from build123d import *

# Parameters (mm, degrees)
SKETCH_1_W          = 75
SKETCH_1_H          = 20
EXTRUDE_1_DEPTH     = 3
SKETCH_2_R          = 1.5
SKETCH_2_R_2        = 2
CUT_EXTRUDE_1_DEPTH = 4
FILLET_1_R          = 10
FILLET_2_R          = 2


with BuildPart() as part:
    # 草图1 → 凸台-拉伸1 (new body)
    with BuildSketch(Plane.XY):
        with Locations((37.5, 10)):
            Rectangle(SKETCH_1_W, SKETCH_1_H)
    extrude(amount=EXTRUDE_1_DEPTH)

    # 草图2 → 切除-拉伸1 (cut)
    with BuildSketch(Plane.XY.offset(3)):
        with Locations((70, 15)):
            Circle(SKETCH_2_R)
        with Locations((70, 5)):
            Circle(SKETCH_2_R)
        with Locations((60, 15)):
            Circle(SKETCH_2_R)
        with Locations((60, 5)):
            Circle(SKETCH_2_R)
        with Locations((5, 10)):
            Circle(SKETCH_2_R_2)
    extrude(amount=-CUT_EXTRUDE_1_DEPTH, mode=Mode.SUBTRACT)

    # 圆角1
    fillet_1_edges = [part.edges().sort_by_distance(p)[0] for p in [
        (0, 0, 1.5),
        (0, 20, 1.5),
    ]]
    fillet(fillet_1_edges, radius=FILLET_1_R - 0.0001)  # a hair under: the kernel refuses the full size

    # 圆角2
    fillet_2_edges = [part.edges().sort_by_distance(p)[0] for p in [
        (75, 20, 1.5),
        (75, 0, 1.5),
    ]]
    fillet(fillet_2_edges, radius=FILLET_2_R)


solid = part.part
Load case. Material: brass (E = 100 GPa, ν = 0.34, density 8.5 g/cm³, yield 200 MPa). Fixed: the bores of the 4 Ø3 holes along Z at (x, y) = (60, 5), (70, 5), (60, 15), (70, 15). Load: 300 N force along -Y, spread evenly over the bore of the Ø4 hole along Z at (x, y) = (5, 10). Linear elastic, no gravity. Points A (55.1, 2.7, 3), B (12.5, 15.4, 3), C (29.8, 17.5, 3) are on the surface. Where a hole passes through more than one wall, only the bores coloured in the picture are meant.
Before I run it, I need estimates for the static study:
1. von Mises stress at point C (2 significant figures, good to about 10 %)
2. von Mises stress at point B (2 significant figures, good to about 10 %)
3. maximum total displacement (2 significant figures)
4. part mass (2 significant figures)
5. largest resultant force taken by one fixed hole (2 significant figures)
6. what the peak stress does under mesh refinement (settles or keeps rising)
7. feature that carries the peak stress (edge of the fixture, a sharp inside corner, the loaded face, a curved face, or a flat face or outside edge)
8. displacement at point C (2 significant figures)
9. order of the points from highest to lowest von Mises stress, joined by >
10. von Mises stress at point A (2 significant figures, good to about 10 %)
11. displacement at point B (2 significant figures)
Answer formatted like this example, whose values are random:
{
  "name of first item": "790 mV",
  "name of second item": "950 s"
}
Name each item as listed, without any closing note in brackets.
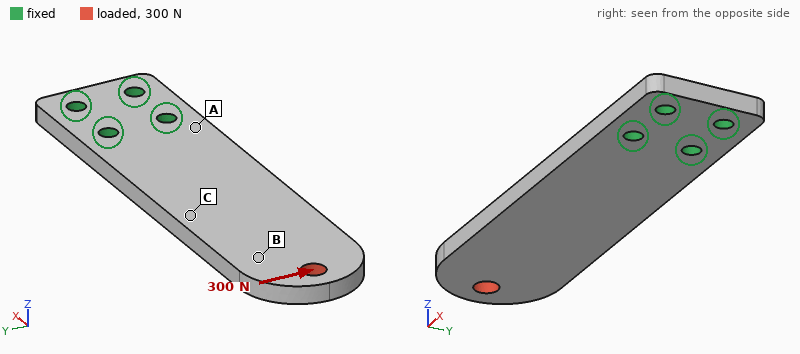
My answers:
{
  "von Mises stress at point C": "29 MPa",
  "von Mises stress at point B": "11 MPa",
  "maximum total displacement": "0.11 mm",
  "part mass": "36 g",
  "largest resultant force taken by one fixed hole": "1.1 kN",
  "what the peak stress does under mesh refinement": "keeps rising",
  "feature that carries the peak stress": "edge of the fixture",
  "displacement at point C": "0.041 mm",
  "order of the points from highest to lowest von Mises stress, joined by >": "A > C > B",
  "von Mises stress at point A": "56 MPa",
  "displacement at point B": "0.080 mm"
}
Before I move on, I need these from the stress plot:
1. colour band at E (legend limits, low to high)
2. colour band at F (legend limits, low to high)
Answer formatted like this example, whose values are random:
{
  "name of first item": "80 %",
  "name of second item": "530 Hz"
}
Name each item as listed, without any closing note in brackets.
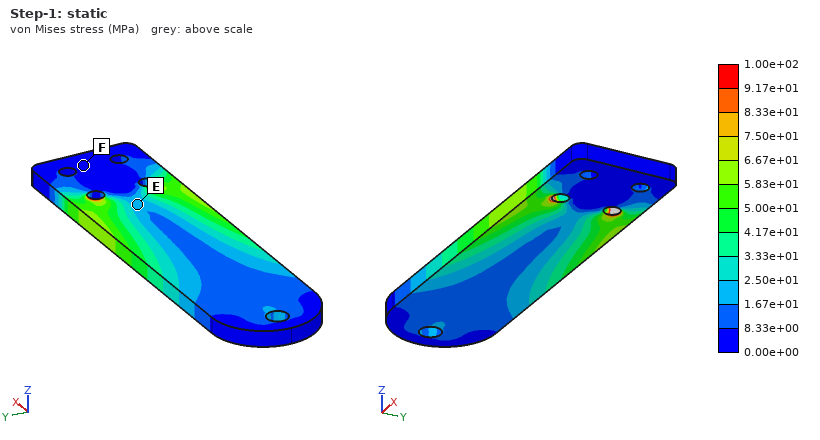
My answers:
{
  "colour band at E": "1.67e+01 to 2.50e+01 MPa",
  "colour band at F": "0.00e+00 to 8.33e+00 MPa"
}
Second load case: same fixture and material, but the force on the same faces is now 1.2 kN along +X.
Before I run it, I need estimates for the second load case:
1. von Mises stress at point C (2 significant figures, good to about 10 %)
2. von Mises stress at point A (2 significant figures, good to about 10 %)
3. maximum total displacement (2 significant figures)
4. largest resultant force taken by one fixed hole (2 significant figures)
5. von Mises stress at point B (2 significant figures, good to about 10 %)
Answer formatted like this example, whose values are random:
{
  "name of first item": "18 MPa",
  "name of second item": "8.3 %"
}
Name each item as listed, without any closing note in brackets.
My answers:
{
  "von Mises stress at point C": "20 MPa",
  "von Mises stress at point A": "20 MPa",
  "maximum total displacement": "14 µm",
  "largest resultant force taken by one fixed hole": "540 N",
  "von Mises stress at point B": "22 MPa"
}
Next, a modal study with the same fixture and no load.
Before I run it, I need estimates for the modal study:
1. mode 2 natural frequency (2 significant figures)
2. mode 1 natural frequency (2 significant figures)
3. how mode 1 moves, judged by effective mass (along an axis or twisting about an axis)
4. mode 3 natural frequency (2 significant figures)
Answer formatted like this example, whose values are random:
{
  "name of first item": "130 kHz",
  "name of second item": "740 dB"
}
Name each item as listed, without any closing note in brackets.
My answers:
{
  "mode 2 natural frequency": "2900 Hz",
  "mode 1 natural frequency": "520 Hz",
  "how mode 1 moves, judged by effective mass": "along Z",
  "mode 3 natural frequency": "3000 Hz"
}
